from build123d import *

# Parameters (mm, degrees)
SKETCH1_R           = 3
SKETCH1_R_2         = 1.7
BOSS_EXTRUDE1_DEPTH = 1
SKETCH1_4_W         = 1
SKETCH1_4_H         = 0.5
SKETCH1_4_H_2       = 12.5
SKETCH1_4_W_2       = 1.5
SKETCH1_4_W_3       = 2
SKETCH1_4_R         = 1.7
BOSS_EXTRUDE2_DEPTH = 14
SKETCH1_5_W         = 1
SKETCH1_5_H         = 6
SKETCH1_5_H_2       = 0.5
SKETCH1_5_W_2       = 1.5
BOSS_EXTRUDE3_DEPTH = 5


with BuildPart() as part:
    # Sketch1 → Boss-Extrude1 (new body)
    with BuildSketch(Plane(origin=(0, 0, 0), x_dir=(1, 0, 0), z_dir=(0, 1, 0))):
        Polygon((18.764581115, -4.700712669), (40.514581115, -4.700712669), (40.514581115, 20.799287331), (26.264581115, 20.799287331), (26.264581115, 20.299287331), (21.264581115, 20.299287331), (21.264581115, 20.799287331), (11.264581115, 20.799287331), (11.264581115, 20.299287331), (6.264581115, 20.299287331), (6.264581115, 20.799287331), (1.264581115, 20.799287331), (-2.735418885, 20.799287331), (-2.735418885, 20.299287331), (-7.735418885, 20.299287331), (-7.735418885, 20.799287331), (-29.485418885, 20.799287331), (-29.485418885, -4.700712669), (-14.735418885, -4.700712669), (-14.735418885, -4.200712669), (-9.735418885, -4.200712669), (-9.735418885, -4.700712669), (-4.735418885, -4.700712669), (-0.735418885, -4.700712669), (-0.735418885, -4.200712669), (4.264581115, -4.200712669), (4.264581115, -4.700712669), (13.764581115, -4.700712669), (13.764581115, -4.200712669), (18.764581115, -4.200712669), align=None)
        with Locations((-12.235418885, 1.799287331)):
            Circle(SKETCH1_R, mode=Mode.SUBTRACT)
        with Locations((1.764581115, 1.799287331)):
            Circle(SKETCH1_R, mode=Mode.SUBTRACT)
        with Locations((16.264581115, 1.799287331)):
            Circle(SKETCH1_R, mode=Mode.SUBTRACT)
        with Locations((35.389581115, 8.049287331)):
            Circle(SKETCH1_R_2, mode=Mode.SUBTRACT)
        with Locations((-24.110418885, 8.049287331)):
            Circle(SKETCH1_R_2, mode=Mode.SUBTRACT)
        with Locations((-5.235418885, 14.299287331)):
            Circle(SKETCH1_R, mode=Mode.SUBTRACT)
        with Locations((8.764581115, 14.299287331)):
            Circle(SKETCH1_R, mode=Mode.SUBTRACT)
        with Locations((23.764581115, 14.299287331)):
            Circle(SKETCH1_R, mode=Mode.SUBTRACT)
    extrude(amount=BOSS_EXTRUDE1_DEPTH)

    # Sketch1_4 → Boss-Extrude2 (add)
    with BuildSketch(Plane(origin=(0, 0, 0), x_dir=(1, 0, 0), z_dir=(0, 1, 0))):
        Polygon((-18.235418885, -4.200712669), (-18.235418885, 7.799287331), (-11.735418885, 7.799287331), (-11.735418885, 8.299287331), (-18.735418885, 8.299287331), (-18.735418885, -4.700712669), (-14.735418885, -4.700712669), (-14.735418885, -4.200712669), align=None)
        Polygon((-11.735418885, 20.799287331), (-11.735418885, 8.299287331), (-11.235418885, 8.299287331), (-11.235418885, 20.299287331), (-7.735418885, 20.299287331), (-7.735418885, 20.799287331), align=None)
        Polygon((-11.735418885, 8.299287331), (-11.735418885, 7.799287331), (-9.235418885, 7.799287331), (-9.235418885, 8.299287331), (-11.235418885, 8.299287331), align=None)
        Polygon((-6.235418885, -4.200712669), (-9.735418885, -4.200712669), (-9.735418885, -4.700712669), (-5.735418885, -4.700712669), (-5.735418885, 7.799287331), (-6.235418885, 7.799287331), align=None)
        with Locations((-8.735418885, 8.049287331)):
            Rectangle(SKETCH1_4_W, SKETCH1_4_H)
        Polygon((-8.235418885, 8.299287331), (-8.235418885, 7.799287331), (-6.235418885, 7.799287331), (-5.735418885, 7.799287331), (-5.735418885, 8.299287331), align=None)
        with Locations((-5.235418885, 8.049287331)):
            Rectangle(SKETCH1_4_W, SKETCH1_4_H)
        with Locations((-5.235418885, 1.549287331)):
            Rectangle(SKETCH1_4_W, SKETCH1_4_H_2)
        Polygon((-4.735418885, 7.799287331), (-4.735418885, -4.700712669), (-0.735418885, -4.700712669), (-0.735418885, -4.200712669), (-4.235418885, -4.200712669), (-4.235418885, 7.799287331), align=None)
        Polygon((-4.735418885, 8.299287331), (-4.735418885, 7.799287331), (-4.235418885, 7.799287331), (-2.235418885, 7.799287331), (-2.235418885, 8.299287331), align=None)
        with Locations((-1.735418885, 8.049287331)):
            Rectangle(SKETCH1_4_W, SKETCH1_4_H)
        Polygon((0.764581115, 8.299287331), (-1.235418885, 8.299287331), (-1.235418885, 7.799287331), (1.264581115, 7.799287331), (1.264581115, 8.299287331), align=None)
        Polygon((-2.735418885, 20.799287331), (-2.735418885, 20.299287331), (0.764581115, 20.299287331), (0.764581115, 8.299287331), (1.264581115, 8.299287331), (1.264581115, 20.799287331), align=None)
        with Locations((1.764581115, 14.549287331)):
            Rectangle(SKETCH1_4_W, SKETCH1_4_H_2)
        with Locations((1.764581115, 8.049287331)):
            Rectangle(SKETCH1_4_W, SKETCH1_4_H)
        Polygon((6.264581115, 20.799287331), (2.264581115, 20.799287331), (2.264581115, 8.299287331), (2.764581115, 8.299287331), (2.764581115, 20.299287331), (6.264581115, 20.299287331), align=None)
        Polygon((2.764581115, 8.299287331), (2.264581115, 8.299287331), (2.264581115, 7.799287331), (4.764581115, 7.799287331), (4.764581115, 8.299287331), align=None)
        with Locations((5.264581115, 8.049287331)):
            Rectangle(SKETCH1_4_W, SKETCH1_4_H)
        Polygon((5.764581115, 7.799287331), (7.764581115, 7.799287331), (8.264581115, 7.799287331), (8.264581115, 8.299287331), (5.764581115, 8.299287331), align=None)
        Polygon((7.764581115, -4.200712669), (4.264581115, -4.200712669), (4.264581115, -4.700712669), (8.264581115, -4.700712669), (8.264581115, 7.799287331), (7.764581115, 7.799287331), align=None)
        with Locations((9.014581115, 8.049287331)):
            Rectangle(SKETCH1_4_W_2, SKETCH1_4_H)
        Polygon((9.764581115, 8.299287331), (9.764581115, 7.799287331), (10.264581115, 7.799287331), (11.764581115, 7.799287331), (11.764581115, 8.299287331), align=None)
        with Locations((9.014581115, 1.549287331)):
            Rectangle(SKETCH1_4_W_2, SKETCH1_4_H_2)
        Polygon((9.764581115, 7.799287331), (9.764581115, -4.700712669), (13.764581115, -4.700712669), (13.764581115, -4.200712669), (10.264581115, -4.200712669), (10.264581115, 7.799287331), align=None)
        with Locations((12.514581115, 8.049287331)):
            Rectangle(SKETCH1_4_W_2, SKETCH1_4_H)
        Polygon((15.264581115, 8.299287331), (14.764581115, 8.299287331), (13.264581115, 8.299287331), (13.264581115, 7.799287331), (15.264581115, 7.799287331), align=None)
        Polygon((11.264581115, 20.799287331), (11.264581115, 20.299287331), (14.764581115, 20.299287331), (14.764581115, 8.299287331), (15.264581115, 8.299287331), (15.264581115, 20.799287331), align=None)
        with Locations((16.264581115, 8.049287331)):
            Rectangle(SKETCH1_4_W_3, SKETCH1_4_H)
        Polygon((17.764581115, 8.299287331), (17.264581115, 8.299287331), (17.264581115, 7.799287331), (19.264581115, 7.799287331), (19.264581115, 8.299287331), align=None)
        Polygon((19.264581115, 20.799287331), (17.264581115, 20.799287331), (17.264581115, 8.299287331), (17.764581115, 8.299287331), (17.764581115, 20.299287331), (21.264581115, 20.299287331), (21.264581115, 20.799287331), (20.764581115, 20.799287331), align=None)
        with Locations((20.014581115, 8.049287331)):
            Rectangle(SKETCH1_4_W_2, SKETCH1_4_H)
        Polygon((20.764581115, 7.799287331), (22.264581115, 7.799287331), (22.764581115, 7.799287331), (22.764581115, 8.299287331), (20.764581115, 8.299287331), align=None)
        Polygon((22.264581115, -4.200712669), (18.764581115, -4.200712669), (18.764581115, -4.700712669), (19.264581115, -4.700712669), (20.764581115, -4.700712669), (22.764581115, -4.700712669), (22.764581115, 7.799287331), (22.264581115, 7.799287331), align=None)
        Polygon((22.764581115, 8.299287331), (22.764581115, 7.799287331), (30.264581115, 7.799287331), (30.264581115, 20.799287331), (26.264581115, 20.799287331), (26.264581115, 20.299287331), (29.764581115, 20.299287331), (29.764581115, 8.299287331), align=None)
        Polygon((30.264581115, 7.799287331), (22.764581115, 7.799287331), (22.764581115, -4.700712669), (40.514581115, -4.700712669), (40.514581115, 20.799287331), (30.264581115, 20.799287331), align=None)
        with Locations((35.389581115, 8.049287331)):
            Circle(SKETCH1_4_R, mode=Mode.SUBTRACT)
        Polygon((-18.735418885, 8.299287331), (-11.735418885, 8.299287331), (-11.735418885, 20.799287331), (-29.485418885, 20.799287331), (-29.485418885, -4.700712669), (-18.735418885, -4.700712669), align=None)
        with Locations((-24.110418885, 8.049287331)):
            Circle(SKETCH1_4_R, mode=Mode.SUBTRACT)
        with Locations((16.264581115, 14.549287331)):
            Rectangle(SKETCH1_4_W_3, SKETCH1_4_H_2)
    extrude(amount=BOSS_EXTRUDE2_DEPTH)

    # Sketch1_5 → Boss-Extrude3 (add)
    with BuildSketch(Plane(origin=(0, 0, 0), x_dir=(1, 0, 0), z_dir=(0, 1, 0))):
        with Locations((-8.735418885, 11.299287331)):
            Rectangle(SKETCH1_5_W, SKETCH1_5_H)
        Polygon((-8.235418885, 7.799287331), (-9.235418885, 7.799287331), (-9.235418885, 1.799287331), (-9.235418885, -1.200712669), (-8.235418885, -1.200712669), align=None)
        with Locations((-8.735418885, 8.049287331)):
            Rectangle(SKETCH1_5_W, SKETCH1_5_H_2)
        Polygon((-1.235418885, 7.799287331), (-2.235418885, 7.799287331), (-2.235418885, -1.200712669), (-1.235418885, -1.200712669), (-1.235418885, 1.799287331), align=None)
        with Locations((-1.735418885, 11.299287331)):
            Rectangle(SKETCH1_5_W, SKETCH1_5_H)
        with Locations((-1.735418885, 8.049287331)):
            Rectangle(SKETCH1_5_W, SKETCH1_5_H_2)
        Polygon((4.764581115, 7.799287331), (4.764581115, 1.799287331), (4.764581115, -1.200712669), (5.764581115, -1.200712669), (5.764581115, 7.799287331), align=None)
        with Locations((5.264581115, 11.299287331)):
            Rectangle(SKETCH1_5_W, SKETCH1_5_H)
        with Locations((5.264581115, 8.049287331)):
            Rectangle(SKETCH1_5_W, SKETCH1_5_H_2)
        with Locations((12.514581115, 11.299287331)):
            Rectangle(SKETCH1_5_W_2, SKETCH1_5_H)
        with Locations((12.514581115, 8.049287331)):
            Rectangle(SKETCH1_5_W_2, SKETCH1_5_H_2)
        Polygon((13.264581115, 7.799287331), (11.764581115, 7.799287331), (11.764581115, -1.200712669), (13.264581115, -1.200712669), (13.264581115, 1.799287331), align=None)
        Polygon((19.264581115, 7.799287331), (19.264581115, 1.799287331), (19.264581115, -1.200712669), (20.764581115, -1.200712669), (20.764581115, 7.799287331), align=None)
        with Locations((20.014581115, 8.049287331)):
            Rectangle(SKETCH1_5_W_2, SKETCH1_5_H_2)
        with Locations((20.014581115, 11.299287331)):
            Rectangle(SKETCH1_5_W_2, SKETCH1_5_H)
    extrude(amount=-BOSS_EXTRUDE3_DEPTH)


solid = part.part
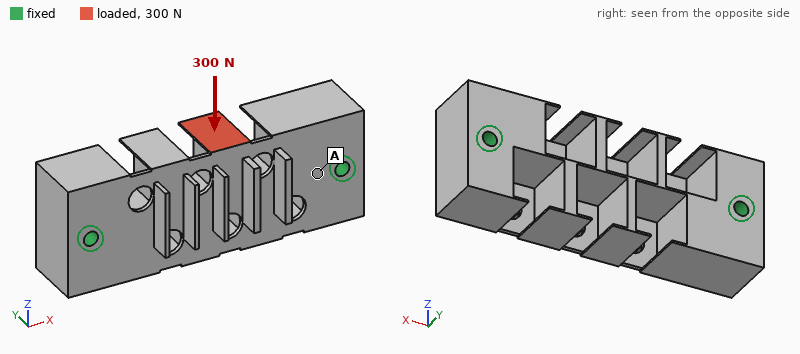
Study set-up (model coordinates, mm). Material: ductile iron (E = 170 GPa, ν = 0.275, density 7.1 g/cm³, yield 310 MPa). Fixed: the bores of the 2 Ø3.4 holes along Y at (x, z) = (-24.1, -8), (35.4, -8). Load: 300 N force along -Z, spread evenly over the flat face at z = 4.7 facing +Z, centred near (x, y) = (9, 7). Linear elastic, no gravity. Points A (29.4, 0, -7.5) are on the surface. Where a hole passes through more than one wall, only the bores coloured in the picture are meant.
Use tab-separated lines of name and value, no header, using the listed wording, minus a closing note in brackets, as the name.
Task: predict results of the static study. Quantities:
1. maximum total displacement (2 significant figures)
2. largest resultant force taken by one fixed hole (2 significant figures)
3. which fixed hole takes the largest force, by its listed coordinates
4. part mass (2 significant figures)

maximum total displacement	70 µm
largest resultant force taken by one fixed hole	180 N
which fixed hole takes the largest force, by its listed coordinates	(35.4, -8)
part mass	96 g
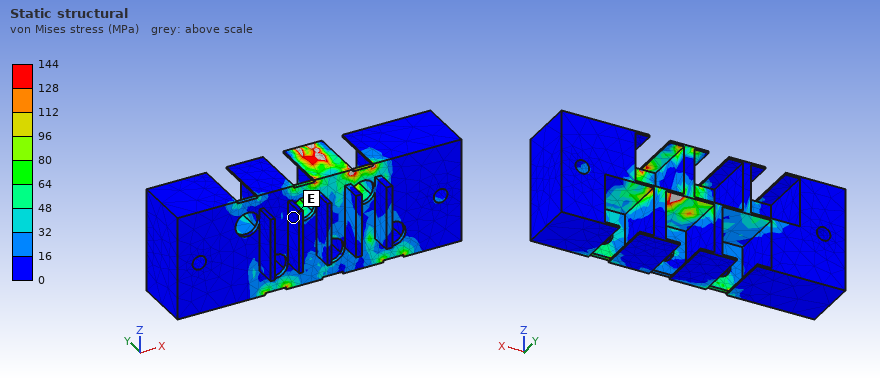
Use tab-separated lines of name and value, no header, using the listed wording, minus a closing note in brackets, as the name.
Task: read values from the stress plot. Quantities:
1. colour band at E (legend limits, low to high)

colour band at E	0 to 16 MPa
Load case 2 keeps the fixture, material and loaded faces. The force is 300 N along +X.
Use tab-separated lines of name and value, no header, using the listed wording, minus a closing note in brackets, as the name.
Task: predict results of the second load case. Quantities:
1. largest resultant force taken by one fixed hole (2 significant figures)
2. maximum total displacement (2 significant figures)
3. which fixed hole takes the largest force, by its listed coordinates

largest resultant force taken by one fixed hole	200 N
maximum total displacement	63 µm
which fixed hole takes the largest force, by its listed coordinates	(35.4, -8)
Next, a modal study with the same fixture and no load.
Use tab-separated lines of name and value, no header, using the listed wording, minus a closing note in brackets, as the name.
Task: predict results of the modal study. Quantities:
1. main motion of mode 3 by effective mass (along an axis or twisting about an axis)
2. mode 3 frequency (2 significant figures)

main motion of mode 3 by effective mass	along Y
mode 3 frequency	7800 Hz
